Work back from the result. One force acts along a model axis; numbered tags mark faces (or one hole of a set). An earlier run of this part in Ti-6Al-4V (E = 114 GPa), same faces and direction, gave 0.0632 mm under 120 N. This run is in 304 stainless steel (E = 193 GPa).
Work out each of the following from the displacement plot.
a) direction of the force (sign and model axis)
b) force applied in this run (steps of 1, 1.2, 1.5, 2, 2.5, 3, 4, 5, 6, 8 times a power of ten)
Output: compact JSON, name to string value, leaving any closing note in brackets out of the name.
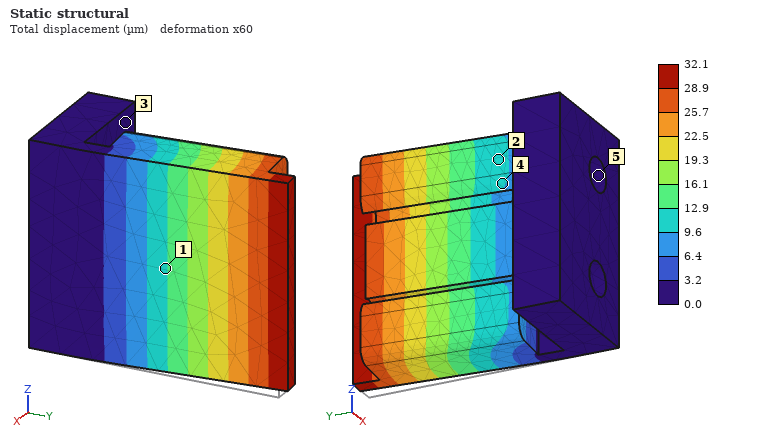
{"direction of the force": "-X", "force applied in this run": "100 N"}
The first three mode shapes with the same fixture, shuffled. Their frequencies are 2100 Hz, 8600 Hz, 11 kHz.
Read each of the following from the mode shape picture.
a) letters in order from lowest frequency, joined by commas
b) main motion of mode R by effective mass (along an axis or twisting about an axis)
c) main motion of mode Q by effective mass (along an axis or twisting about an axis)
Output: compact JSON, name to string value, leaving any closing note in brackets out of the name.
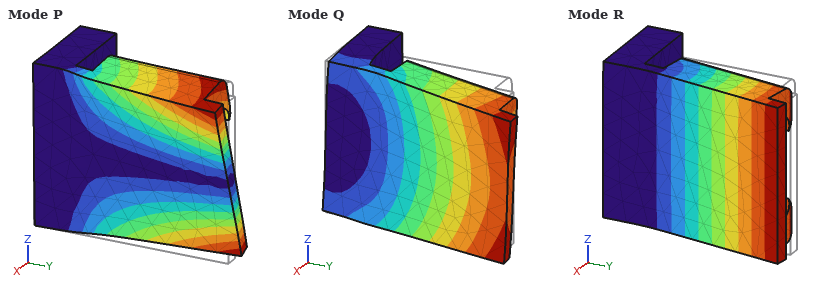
{"letters in order from lowest frequency, joined by commas": "R, P, Q", "main motion of mode R by effective mass": "along X", "main motion of mode Q by effective mass": "along Z"}
